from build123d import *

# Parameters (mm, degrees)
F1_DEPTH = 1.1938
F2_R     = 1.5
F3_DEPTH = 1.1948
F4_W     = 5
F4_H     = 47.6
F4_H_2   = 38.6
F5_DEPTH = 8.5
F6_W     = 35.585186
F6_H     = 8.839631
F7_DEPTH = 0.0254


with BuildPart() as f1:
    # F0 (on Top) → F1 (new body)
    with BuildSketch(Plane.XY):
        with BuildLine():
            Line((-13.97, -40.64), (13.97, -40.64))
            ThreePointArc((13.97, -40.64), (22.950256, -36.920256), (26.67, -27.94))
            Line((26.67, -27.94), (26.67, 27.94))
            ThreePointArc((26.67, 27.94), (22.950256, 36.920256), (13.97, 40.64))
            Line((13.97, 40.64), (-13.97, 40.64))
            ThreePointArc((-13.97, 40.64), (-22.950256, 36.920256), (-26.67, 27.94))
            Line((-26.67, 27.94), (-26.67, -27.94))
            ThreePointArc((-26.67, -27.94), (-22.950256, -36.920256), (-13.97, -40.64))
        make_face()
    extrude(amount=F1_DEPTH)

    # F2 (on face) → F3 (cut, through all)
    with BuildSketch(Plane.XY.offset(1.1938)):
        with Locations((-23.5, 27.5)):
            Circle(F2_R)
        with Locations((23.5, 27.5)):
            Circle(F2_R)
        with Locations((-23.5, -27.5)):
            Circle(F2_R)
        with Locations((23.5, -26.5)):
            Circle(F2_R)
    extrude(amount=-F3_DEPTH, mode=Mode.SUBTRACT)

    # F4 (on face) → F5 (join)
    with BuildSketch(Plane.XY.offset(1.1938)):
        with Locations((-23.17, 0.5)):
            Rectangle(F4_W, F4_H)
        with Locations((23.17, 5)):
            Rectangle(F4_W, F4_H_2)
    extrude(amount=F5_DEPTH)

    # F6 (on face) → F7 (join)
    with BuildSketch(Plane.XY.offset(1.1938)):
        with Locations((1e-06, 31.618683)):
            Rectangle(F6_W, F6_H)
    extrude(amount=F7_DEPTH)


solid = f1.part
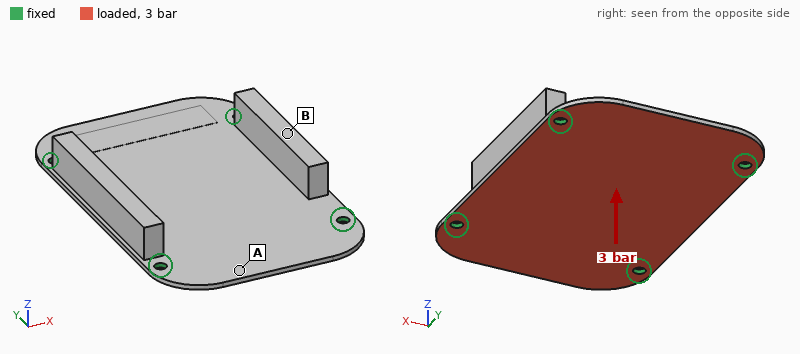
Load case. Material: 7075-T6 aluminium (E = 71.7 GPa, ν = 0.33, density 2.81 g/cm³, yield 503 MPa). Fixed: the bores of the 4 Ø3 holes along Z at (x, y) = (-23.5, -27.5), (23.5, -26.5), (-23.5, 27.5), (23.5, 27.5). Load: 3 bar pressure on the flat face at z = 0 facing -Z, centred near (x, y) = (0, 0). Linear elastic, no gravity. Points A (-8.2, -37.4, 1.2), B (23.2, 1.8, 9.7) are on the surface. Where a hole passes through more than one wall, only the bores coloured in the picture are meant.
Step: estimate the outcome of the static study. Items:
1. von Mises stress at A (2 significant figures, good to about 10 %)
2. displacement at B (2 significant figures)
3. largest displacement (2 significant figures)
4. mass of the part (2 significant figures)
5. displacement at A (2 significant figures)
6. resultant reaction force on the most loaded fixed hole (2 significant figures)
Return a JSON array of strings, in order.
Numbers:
["89 MPa", "0.21 mm", "0.59 mm", "24 g", "0.45 mm", "360 N"]
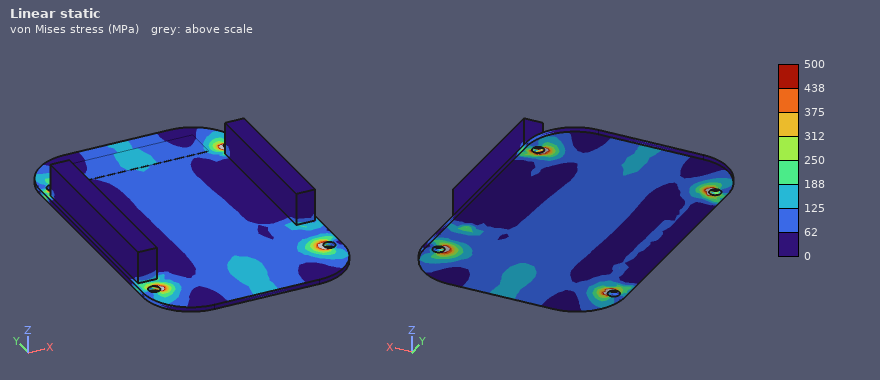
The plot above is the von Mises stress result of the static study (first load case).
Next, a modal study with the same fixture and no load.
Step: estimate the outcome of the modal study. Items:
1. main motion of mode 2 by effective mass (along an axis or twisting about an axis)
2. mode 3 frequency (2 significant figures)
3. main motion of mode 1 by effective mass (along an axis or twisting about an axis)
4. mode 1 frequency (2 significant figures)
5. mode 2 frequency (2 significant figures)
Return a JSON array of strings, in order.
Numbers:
["twisting about X", "2800 Hz", "along Z", "2300 Hz", "2600 Hz"]
